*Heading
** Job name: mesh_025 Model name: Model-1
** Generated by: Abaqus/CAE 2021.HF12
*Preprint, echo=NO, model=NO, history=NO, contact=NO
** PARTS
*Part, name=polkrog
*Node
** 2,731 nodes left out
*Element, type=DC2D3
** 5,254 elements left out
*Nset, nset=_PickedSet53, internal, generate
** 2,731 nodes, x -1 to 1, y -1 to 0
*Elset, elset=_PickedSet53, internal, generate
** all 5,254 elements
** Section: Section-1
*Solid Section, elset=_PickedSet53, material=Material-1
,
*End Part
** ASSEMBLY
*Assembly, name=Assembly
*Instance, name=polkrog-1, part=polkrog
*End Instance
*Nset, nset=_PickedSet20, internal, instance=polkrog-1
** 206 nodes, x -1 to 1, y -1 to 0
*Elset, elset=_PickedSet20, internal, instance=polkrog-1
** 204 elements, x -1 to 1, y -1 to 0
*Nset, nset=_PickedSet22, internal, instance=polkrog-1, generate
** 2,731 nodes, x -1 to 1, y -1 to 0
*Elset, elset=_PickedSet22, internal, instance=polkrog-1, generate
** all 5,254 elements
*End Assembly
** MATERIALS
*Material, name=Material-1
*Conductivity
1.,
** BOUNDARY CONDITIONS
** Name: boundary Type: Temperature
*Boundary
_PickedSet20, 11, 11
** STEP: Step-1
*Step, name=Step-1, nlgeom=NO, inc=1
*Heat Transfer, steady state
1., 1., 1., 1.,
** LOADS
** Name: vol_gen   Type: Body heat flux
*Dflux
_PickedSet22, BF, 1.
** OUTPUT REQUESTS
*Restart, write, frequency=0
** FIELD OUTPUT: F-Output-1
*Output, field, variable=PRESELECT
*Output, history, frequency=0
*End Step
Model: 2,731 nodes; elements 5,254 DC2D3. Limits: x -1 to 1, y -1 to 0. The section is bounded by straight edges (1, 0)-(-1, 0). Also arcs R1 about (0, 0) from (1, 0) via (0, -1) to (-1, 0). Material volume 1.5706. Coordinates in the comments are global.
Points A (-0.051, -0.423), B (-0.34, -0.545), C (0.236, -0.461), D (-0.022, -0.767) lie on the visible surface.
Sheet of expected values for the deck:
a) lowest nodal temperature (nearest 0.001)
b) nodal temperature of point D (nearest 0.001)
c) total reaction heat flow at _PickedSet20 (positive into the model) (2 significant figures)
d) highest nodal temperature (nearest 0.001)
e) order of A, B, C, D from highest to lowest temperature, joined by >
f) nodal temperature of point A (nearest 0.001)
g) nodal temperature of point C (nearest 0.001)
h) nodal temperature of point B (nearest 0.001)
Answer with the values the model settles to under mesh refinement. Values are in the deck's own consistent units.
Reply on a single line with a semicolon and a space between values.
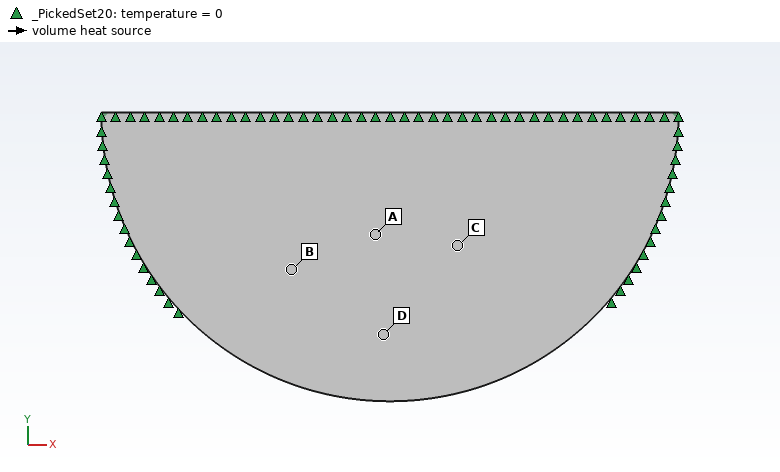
0.000; 0.067; -1.6; 0.098; A > C > B > D; 0.096; 0.091; 0.082
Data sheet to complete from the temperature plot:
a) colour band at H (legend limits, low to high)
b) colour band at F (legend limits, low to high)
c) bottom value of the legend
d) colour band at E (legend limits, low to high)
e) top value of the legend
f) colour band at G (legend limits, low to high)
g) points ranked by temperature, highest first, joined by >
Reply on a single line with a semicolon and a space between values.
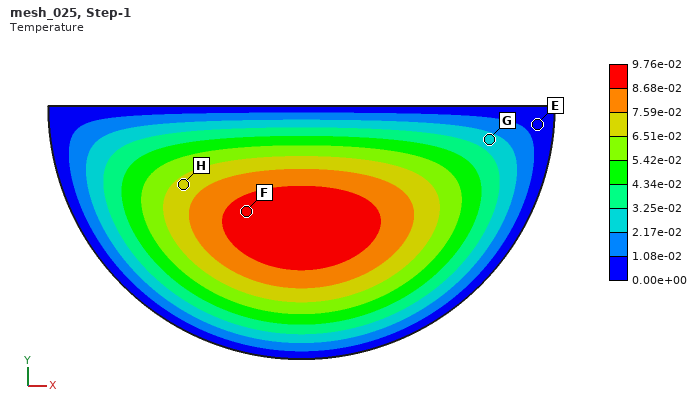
6.51e-02 to 7.59e-02; 8.68e-02 to 9.76e-02; 0.00e+00; 0.00e+00 to 1.08e-02; 9.76e-02; 2.17e-02 to 3.25e-02; F > H > G > E
